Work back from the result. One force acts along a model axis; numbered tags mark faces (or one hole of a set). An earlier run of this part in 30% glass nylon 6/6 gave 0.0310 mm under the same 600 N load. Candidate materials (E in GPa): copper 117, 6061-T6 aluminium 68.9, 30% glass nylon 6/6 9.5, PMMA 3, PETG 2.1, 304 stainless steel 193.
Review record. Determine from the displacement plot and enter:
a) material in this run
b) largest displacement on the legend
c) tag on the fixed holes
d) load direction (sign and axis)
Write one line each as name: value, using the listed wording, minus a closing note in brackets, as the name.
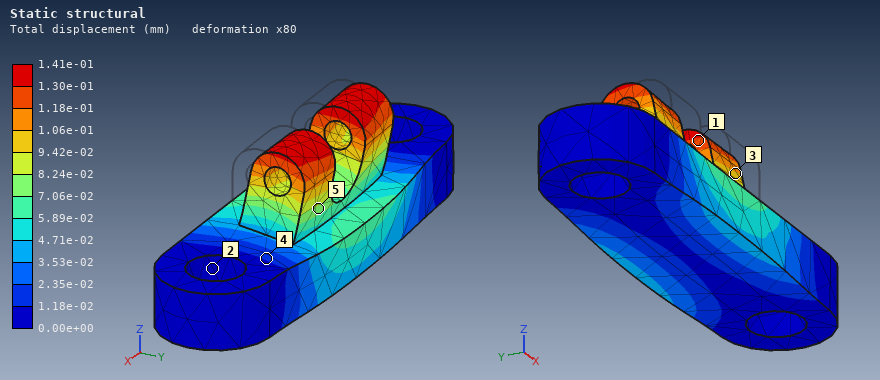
material in this run: PETG
largest displacement on the legend: 1.41e-01 mm
tag on the fixed holes: 2
load direction: +Y
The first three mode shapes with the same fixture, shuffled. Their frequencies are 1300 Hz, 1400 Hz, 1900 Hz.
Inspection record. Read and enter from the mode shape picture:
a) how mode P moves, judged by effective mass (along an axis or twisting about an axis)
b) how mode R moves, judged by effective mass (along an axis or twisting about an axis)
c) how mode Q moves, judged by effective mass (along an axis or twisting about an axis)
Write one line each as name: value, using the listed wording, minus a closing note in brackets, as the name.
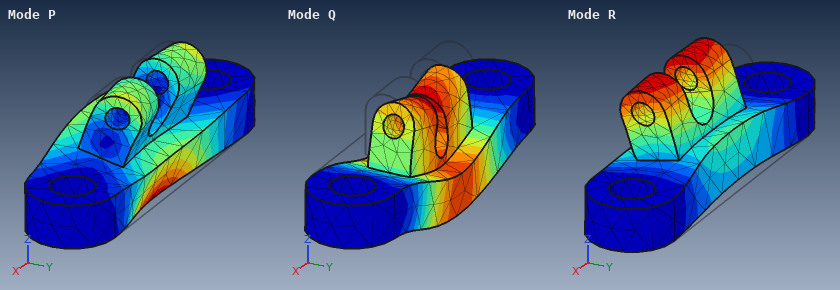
how mode P moves, judged by effective mass: along Y
how mode R moves, judged by effective mass: along Y
how mode Q moves, judged by effective mass: along Z
